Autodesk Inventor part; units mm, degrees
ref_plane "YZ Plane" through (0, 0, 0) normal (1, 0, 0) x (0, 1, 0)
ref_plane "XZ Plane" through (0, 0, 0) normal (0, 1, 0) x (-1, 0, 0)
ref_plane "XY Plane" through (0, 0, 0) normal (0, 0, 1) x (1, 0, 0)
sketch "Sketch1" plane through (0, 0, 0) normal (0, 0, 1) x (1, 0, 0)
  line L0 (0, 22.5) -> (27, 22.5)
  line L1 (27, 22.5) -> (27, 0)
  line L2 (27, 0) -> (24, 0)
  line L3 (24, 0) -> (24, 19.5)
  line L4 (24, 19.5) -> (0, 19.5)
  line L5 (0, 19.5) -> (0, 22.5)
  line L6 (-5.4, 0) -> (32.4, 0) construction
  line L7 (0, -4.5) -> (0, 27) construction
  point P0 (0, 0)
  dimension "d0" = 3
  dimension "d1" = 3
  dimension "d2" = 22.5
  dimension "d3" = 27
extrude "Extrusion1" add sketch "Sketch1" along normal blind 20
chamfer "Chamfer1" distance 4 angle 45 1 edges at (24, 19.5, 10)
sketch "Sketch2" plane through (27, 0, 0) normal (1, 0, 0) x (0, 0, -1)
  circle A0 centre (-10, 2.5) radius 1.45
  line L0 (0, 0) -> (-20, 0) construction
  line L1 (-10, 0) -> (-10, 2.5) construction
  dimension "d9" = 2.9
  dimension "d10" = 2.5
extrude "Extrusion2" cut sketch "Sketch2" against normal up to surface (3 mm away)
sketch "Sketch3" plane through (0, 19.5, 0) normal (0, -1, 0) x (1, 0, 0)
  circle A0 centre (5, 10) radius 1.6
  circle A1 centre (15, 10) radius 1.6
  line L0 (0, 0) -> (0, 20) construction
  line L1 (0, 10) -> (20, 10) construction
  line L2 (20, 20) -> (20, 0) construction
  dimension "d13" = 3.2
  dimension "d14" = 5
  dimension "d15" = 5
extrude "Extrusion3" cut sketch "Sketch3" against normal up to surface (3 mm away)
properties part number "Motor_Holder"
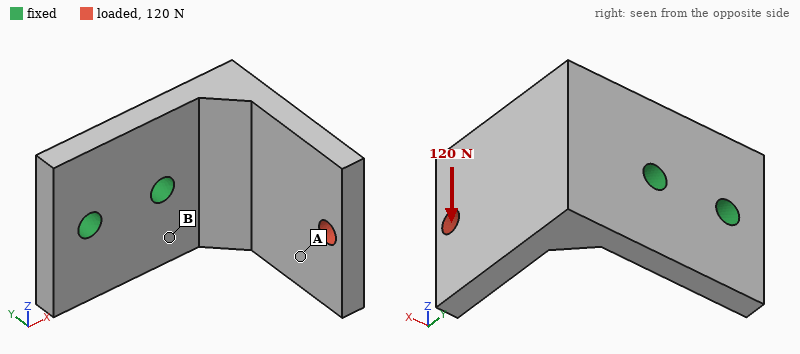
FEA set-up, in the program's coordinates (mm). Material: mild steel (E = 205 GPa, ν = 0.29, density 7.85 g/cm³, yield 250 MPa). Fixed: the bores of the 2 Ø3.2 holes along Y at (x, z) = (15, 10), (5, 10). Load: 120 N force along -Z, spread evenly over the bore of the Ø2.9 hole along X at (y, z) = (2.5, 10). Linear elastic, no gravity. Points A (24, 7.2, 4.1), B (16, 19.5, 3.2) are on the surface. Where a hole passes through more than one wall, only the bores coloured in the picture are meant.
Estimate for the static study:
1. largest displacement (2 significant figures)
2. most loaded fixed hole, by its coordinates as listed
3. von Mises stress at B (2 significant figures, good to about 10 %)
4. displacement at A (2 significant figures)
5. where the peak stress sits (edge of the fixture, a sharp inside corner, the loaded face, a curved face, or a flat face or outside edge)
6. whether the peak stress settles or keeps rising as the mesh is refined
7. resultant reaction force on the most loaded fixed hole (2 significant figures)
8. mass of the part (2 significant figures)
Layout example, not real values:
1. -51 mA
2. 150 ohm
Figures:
1. 24 µm
2. (15, 10)
3. 25 MPa
4. 16 µm
5. edge of the fixture
6. keeps rising
7. 200 N
8. 23 g
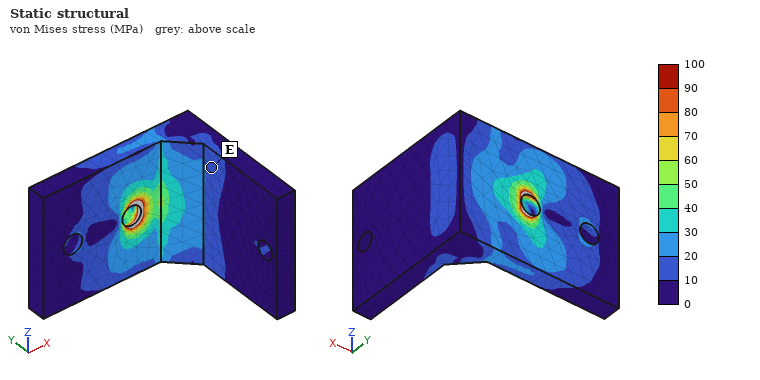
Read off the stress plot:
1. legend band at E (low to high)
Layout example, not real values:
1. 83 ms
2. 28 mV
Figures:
1. 10 to 20 MPa
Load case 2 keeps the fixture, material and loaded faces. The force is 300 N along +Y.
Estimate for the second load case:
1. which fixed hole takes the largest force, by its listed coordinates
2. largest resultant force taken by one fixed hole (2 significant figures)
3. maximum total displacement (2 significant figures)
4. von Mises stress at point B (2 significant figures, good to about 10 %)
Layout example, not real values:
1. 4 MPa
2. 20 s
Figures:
1. (15, 10)
2. 400 N
3. 38 µm
4. 50 MPa
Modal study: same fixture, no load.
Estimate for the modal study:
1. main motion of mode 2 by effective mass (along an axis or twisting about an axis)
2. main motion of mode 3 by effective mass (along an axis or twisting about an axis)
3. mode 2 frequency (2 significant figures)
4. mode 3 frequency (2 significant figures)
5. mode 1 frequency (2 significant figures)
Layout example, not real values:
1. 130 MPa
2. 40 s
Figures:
1. along Z
2. along Y
3. 5400 Hz
4. 12 kHz
5. 3800 Hz
